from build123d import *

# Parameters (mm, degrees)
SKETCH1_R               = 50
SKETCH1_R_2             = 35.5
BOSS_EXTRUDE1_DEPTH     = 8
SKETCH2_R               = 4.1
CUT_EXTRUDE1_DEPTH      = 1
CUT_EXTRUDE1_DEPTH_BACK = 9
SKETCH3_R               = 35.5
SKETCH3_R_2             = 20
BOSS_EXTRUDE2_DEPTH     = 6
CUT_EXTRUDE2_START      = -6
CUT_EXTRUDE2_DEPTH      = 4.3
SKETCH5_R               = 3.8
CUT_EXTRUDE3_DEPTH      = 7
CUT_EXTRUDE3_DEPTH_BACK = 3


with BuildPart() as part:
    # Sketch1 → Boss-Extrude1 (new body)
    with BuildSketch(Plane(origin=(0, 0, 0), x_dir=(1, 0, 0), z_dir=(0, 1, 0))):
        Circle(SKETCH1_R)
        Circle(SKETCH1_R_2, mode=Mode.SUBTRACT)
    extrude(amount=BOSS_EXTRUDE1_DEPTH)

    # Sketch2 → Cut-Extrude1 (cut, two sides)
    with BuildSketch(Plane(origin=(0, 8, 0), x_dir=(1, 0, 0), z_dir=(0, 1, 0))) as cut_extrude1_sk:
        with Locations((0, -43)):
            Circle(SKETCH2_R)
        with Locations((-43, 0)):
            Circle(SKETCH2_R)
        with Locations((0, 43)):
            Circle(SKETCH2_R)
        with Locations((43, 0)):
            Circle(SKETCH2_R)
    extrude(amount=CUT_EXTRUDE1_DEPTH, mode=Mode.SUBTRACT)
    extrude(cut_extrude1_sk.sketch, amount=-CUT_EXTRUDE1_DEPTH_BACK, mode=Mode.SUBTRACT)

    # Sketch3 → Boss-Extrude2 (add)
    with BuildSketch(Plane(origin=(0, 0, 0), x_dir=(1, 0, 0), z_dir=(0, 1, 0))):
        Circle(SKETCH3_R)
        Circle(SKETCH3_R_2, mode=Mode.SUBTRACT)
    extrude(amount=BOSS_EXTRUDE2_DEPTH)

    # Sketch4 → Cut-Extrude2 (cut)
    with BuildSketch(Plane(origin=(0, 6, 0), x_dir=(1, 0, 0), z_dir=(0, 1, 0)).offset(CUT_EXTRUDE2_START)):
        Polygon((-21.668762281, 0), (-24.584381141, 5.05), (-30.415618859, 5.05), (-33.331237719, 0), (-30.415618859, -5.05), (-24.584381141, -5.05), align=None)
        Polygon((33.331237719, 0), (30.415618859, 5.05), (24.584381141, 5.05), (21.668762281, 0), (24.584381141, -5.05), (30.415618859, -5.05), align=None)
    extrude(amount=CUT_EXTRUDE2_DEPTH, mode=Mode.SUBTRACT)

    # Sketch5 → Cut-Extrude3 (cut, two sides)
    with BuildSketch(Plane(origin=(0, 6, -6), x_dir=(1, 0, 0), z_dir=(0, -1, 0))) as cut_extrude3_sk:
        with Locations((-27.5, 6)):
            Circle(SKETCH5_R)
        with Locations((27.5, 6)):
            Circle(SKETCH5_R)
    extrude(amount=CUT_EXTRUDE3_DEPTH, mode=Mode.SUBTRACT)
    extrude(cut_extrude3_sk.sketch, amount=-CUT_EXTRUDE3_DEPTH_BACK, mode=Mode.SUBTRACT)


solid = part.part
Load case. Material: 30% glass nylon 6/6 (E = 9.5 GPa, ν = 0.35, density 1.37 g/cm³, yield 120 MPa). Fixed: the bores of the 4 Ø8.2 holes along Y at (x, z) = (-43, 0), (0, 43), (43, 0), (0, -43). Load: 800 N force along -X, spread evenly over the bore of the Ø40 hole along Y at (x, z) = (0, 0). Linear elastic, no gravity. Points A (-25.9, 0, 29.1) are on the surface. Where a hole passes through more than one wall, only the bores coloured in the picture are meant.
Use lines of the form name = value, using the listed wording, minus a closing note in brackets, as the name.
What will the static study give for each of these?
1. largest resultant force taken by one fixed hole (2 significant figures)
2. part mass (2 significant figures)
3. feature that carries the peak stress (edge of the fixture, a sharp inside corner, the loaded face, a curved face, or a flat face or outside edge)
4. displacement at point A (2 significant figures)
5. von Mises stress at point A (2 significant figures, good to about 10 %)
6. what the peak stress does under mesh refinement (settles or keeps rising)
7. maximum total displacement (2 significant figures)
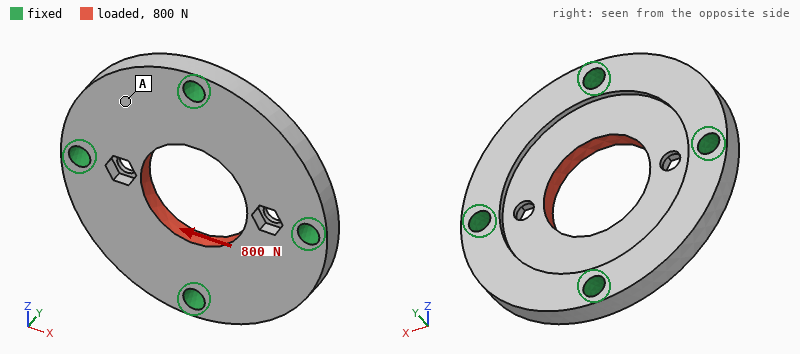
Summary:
largest resultant force taken by one fixed hole = 210 N
part mass = 61 g
feature that carries the peak stress = a sharp inside corner
displacement at point A = 4.1 µm
von Mises stress at point A = 0.50 MPa
what the peak stress does under mesh refinement = keeps rising
maximum total displacement = 9.6 µm
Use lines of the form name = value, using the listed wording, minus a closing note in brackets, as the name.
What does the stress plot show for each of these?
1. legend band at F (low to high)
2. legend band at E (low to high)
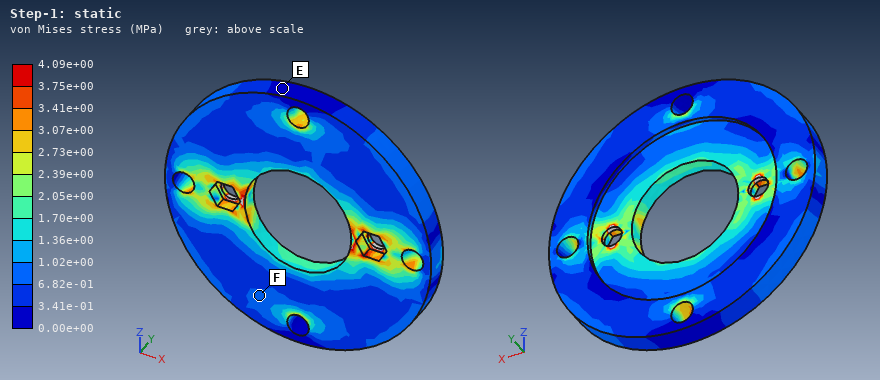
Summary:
legend band at F = 6.82e-01 to 1.02e+00 MPa
legend band at E = 0.00e+00 to 3.41e-01 MPa
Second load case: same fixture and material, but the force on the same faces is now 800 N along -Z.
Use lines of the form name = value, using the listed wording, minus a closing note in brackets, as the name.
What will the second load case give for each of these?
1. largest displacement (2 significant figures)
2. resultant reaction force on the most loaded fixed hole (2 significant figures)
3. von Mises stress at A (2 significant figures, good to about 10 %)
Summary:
largest displacement = 5.8 µm
resultant reaction force on the most loaded fixed hole = 240 N
von Mises stress at A = 0.46 MPa
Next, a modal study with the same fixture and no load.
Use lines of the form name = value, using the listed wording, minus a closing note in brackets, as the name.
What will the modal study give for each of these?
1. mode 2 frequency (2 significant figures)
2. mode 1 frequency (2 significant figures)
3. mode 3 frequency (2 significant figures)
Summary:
mode 2 frequency = 4800 Hz
mode 1 frequency = 4700 Hz
mode 3 frequency = 4900 Hz
